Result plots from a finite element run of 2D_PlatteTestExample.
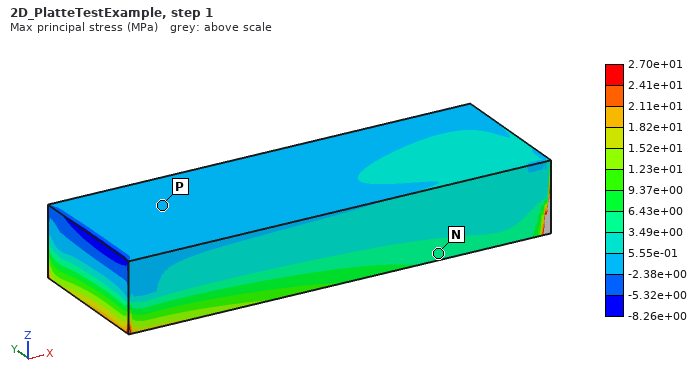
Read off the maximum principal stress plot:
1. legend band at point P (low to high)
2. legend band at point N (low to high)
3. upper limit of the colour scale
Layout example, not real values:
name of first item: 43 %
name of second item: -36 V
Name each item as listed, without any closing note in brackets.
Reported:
legend band at point P: -2.38e+00 to 5.55e-01 MPa
legend band at point N: 3.49e+00 to 6.43e+00 MPa
upper limit of the colour scale: 2.70e+01 MPa
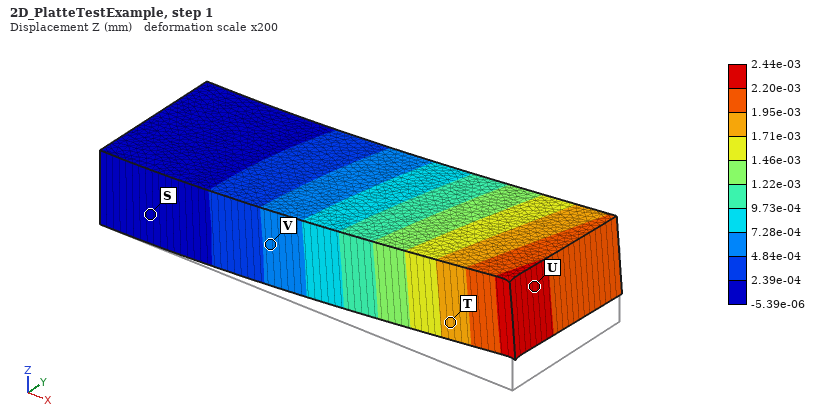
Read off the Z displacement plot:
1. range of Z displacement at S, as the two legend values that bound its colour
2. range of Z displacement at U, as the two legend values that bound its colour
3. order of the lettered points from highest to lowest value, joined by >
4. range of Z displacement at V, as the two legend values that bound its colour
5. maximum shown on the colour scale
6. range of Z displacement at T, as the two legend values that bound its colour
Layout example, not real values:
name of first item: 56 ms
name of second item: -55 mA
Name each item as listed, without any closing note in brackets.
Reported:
range of Z displacement at S, as the two legend values that bound its colour: -5.39e-06 to 2.39e-04 mm
range of Z displacement at U, as the two legend values that bound its colour: 2.20e-03 to 2.44e-03 mm
order of the lettered points from highest to lowest value, joined by >: U > T > V > S
range of Z displacement at V, as the two legend values that bound its colour: 4.84e-04 to 7.28e-04 mm
maximum shown on the colour scale: 2.44e-03 mm
range of Z displacement at T, as the two legend values that bound its colour: 1.71e-03 to 1.95e-03 mm
